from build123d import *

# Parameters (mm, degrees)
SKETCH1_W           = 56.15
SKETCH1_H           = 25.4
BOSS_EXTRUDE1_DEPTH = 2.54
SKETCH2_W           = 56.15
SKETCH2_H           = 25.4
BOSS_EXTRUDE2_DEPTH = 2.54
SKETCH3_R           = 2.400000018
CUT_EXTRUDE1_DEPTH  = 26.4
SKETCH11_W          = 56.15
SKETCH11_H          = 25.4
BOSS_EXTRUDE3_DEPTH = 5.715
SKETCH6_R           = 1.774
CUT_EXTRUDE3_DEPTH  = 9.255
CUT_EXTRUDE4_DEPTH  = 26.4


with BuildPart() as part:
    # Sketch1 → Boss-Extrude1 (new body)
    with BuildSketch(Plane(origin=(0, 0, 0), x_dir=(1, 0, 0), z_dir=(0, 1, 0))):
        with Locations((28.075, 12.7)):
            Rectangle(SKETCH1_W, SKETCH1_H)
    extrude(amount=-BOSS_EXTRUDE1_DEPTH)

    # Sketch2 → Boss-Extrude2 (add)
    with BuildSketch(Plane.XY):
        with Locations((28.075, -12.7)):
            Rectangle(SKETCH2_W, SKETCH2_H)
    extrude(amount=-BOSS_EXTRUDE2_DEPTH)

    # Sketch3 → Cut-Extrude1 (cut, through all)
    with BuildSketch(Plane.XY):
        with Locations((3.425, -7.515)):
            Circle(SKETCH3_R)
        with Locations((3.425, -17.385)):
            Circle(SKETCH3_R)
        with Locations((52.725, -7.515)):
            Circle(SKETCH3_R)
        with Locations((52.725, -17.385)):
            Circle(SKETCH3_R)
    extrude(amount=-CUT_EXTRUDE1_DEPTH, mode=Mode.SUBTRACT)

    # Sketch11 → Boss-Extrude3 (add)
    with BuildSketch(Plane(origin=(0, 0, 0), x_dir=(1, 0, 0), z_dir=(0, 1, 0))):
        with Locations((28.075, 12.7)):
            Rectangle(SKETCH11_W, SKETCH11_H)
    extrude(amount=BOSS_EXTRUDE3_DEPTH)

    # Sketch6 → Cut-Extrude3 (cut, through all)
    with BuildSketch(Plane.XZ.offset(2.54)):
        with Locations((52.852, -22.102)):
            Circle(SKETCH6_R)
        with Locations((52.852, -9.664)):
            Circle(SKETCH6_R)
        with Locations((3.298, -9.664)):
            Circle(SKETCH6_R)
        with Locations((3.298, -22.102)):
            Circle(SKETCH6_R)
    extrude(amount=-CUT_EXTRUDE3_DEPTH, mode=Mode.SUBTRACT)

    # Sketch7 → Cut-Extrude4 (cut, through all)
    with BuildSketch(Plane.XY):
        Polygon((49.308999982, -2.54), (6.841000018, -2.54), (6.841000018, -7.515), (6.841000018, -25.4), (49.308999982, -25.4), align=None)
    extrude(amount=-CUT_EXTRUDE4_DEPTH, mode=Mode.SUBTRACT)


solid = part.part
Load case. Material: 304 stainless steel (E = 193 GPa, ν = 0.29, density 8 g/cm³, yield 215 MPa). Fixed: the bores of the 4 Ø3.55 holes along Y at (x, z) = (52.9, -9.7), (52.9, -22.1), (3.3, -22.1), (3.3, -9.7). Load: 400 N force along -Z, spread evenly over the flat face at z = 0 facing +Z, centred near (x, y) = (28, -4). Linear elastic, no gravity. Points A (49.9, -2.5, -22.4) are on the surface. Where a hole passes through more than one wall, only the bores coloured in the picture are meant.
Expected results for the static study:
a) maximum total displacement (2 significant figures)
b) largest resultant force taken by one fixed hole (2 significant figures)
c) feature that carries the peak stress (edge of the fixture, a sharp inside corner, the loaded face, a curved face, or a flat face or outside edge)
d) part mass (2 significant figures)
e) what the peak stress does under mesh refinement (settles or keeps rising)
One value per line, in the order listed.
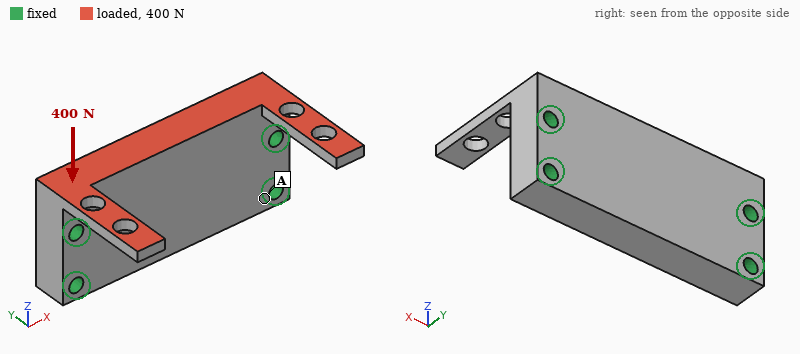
0.14 mm
160 N
a sharp inside corner
96 g
keeps rising
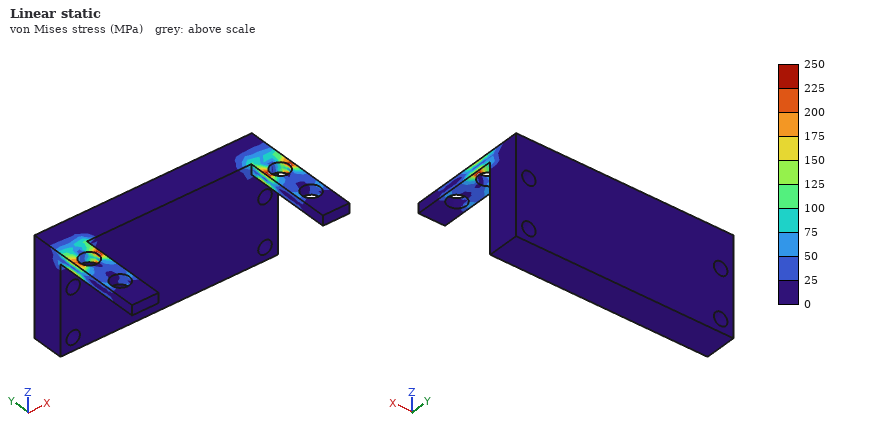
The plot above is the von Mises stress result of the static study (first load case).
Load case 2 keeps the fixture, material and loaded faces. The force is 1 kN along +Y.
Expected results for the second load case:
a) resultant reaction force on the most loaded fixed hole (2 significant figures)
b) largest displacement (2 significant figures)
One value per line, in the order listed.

590 N
52 µm
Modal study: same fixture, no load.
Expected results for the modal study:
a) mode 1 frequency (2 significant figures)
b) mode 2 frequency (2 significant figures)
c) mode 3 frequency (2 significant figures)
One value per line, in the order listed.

2800 Hz
2800 Hz
6900 Hz
